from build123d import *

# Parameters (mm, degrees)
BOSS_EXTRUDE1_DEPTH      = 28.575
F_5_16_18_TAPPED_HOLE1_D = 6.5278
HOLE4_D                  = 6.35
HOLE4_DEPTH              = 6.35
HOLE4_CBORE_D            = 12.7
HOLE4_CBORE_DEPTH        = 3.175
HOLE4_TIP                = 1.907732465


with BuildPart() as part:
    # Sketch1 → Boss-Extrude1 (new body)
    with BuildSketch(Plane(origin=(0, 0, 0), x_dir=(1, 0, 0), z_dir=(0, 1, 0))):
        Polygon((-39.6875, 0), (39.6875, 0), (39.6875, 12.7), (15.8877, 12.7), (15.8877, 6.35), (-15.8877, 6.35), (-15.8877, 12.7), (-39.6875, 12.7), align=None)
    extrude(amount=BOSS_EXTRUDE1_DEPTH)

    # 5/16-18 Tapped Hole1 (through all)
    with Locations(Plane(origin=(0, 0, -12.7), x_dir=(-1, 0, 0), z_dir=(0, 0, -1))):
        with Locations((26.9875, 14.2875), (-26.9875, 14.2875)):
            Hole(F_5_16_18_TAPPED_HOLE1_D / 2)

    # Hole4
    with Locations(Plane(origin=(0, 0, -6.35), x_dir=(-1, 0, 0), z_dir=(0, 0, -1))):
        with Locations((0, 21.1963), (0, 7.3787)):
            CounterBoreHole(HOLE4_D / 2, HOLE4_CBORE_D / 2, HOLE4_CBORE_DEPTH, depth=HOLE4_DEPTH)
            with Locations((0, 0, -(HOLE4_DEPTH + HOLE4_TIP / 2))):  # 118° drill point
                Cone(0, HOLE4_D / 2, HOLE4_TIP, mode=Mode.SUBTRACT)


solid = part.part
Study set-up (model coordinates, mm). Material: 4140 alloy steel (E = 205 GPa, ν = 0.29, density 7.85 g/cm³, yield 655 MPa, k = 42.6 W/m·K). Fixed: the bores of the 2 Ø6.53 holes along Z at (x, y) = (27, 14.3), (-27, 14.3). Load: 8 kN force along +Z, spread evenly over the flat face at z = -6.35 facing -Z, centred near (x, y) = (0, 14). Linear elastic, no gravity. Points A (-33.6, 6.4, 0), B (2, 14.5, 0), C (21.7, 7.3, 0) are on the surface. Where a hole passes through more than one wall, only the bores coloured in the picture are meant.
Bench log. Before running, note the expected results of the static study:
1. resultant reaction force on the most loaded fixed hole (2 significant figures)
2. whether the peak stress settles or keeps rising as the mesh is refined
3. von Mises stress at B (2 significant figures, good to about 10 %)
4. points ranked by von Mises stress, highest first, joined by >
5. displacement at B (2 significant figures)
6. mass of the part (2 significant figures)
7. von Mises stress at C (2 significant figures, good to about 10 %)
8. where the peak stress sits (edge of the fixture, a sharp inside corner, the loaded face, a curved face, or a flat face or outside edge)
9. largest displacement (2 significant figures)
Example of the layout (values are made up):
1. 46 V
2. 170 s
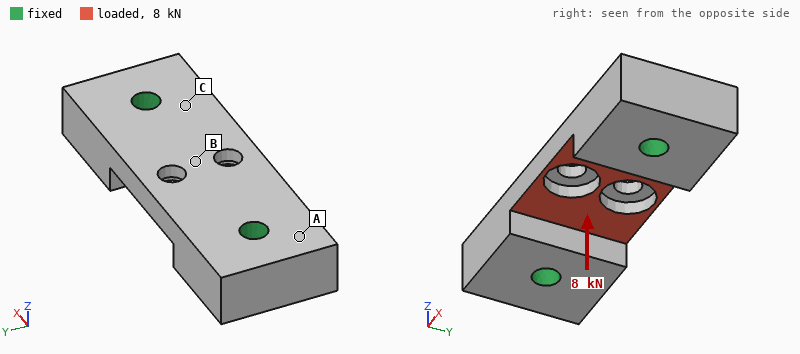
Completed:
1. 4.5 kN
2. keeps rising
3. 94 MPa
4. B > C > A
5. 18 µm
6. 170 g
7. 41 MPa
8. edge of the fixture
9. 21 µm
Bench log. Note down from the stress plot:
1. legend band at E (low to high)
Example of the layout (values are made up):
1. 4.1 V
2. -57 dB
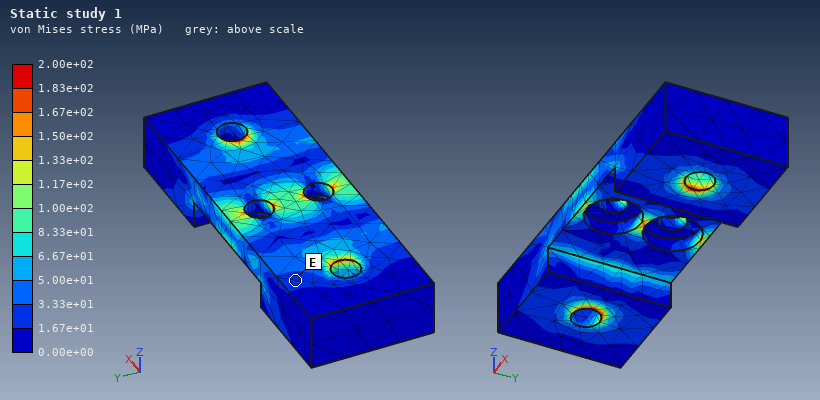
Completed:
1. 1.67e+01 to 3.33e+01 MPa
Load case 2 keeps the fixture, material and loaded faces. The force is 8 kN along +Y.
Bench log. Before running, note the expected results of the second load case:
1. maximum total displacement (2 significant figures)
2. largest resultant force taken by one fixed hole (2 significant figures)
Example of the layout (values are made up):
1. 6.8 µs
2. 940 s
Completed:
1. 11 µm
2. 4.0 kN
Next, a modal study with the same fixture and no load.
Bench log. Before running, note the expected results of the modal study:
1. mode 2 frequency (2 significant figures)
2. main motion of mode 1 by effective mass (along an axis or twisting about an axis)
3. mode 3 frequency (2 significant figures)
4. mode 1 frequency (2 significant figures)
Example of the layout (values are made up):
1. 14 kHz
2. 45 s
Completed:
1. 19 kHz
2. along Z
3. 23 kHz
4. 18 kHz
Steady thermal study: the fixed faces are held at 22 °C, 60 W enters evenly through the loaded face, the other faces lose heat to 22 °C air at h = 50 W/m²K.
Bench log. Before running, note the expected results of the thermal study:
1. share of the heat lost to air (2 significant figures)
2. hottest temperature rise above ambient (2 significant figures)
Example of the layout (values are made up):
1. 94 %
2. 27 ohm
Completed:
1. 9.8 %
2. 54 K
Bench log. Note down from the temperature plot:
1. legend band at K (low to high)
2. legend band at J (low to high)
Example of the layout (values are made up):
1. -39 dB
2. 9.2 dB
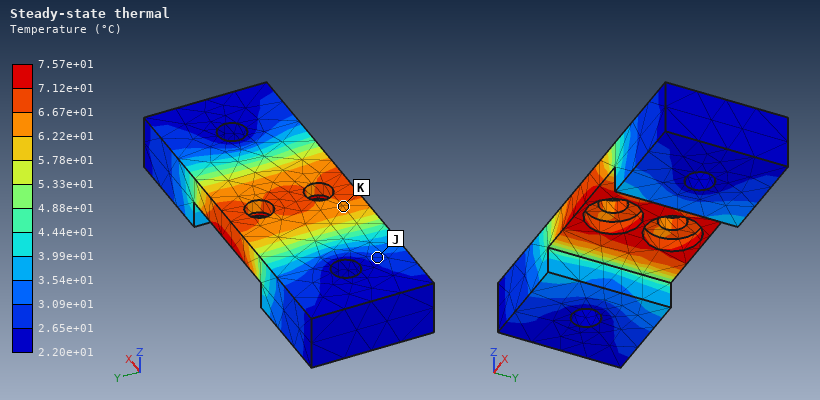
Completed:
1. 6.22e+01 to 6.67e+01 °C
2. 2.65e+01 to 3.09e+01 °C
